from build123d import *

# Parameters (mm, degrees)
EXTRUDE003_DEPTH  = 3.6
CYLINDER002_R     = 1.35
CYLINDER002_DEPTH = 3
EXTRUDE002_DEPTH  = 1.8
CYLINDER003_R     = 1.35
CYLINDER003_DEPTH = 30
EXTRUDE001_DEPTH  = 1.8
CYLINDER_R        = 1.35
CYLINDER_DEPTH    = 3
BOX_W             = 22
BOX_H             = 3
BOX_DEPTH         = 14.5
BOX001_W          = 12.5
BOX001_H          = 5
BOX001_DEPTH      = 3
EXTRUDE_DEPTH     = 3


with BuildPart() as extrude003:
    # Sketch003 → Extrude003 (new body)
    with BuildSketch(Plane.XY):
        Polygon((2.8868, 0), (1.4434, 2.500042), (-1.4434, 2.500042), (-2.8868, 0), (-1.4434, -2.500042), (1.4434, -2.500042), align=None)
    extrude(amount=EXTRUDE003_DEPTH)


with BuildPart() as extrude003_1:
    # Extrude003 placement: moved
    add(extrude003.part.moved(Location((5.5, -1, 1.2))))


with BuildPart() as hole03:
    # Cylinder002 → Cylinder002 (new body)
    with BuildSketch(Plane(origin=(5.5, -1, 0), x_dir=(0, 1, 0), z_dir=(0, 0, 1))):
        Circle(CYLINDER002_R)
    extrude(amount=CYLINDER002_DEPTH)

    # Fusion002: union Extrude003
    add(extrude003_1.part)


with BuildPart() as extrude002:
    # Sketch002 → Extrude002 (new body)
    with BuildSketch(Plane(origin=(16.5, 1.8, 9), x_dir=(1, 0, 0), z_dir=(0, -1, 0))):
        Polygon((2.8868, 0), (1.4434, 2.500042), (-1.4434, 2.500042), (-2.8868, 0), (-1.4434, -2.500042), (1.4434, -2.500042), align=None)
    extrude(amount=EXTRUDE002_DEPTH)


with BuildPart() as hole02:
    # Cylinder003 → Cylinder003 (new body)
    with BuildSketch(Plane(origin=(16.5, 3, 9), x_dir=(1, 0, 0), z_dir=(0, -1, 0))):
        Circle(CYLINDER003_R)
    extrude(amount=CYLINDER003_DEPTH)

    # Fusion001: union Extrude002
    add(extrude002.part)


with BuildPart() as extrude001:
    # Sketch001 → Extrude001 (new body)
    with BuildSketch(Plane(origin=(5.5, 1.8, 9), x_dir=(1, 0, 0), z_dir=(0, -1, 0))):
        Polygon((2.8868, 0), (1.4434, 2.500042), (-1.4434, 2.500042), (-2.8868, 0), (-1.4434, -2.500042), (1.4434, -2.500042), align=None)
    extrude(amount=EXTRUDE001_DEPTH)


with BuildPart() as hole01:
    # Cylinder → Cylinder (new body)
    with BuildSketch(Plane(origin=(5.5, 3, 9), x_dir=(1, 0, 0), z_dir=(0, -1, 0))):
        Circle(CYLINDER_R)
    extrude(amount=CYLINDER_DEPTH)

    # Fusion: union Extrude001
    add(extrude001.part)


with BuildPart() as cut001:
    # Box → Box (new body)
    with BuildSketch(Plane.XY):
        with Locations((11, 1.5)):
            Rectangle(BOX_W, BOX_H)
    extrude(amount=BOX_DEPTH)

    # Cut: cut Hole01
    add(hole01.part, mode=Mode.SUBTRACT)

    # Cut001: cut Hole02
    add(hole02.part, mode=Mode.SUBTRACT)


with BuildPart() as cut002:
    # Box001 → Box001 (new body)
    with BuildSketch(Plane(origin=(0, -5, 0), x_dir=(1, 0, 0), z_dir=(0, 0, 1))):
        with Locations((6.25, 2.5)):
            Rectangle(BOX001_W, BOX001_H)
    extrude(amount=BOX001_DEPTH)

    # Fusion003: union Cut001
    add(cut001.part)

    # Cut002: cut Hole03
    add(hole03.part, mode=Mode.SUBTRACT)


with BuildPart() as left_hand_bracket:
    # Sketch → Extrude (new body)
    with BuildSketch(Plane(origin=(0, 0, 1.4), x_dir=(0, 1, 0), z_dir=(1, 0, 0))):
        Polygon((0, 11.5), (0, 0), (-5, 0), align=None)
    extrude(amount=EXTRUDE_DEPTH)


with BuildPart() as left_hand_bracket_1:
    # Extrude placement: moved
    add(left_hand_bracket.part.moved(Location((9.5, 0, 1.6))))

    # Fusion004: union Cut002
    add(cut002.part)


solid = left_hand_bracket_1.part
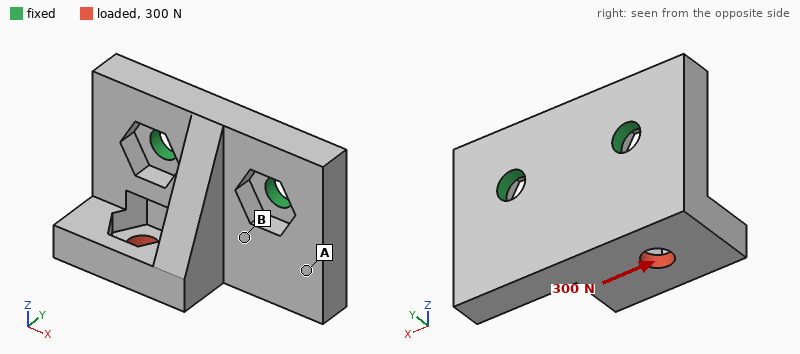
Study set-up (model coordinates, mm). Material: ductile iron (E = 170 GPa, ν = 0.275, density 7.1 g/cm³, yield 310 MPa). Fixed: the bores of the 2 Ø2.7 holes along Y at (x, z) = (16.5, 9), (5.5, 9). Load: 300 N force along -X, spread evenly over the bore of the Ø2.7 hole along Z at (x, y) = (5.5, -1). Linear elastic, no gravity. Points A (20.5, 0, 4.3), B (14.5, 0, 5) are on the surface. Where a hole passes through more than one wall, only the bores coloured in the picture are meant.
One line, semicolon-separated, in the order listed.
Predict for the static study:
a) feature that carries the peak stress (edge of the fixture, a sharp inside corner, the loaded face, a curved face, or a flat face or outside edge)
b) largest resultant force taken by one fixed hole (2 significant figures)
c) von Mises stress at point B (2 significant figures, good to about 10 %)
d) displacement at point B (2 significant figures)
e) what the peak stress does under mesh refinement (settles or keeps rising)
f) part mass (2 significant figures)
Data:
edge of the fixture; 280 N; 18 MPa; 0.99 µm; keeps rising; 7.7 g
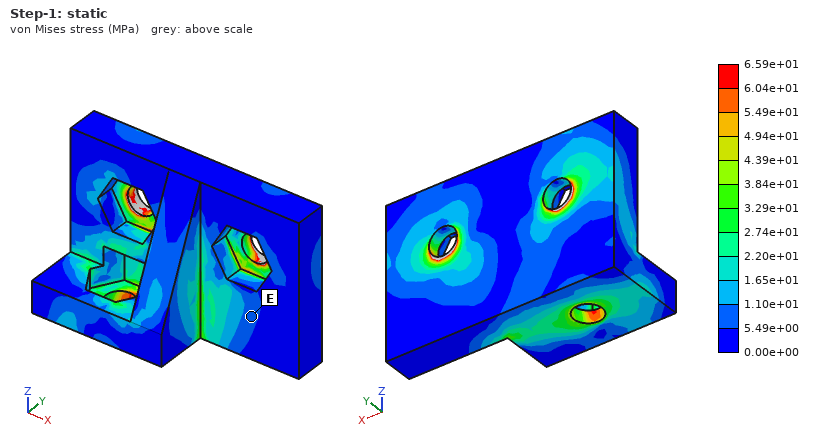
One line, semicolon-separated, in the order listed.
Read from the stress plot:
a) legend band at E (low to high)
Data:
5.49e+00 to 1.10e+01 MPa
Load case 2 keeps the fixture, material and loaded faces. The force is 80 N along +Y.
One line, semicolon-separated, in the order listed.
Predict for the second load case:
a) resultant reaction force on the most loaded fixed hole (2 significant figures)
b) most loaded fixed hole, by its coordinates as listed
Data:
78 N; (5.5, 9)
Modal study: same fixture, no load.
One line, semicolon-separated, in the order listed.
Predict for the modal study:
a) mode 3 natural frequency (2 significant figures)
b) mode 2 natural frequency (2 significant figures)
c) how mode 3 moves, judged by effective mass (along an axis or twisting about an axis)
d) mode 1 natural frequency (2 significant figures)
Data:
32 kHz; 21 kHz; along X; 11 kHz
